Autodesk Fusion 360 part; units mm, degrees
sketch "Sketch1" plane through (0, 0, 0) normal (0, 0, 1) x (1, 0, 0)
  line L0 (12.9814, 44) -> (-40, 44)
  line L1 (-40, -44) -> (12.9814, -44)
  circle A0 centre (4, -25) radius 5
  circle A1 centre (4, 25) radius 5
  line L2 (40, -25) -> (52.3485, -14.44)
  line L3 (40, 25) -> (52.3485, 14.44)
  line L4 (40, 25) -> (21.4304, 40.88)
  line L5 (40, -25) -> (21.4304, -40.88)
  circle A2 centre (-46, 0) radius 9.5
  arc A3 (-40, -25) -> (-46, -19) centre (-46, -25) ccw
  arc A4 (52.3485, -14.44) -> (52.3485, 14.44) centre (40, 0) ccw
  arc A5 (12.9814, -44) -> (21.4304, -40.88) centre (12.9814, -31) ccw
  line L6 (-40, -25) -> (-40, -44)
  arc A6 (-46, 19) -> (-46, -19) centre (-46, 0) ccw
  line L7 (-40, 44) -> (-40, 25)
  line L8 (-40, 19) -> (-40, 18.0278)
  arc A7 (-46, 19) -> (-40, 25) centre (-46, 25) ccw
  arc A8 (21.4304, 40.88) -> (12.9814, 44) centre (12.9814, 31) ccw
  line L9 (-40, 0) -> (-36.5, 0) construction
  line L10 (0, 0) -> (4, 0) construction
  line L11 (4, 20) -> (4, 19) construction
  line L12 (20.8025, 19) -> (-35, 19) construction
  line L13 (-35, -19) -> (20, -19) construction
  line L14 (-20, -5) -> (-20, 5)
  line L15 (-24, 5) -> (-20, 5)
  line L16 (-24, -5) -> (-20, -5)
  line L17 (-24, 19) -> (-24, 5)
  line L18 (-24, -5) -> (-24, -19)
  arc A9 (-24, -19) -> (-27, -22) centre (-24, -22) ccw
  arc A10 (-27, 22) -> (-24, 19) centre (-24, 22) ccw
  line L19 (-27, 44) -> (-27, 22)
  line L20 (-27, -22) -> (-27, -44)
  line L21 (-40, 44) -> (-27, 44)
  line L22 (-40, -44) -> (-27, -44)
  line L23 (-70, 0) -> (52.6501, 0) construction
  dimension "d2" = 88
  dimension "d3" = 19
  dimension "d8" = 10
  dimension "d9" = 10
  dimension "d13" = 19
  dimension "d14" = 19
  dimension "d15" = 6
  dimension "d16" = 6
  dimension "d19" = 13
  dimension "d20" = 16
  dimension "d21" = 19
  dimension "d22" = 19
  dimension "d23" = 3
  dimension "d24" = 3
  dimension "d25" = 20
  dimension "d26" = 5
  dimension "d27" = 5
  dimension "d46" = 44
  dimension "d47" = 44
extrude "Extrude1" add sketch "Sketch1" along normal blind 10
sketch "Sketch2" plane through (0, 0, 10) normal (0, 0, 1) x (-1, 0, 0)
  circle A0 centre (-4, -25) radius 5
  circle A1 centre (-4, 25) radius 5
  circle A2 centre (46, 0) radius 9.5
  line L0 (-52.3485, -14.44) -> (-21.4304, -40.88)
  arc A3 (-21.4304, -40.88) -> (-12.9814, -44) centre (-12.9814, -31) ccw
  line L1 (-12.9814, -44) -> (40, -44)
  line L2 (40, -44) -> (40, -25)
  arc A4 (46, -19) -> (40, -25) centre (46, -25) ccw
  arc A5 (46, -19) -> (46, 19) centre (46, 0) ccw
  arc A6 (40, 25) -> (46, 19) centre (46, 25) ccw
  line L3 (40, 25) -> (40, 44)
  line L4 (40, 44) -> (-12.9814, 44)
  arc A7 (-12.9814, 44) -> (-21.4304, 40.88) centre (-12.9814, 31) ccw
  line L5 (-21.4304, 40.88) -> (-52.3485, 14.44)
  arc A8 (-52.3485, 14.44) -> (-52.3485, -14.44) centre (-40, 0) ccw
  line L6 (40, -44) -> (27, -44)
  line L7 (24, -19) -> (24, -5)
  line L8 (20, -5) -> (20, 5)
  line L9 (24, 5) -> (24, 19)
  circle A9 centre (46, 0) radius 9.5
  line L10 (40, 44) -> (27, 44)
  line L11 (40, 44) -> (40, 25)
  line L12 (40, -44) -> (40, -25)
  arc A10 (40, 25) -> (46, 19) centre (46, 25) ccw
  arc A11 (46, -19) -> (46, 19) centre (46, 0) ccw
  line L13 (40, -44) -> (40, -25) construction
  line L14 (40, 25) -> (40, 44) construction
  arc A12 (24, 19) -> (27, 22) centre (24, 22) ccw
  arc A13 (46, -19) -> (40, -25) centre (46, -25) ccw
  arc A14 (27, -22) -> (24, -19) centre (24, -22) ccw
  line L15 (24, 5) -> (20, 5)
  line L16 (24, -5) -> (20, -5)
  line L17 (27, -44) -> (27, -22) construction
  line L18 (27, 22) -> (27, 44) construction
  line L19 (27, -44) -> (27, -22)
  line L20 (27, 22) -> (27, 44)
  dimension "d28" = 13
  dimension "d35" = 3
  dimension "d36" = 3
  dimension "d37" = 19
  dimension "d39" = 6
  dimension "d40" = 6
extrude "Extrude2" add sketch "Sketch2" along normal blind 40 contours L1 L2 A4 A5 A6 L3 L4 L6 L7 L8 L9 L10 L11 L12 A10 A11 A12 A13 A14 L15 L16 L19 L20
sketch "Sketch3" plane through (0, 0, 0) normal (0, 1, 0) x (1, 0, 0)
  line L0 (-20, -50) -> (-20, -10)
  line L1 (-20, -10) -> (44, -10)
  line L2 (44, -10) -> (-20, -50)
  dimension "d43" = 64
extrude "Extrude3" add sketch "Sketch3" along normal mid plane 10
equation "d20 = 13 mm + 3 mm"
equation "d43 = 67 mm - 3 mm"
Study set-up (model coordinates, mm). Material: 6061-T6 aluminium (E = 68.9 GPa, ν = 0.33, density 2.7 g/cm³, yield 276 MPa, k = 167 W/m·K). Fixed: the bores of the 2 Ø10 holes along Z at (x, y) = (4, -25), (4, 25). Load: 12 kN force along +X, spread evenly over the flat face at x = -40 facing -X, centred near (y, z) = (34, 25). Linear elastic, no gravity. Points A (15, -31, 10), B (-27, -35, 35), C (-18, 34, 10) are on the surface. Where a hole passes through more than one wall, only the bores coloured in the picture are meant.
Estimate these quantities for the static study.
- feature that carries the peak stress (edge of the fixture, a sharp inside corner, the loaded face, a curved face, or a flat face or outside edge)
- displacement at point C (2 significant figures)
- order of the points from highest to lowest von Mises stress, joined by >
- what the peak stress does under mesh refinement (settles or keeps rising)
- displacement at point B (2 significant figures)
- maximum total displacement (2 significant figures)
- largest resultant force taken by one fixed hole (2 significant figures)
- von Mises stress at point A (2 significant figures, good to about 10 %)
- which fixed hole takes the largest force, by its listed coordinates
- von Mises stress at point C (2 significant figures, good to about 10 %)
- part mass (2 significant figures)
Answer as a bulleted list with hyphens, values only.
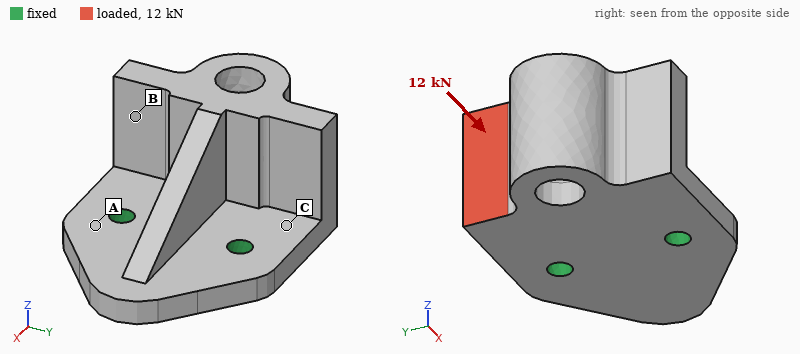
- edge of the fixture
- 0.071 mm
- C > A > B
- keeps rising
- 0.14 mm
- 0.39 mm
- 14 kN
- 50 MPa
- (4, 25)
- 93 MPa
- 440 g
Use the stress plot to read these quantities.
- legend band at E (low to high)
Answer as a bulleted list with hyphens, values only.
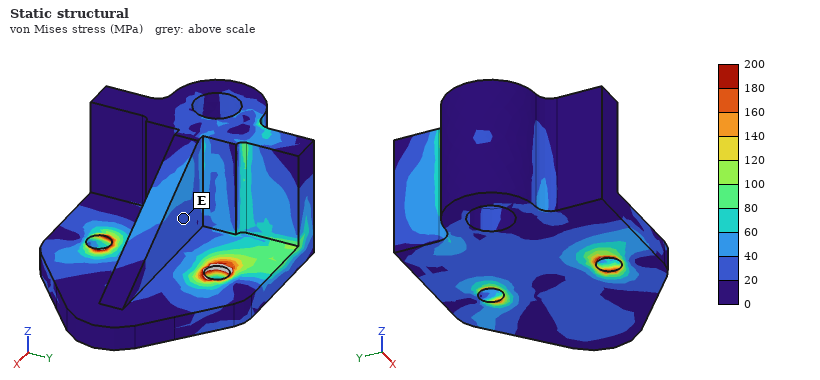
- 20 to 40 MPa
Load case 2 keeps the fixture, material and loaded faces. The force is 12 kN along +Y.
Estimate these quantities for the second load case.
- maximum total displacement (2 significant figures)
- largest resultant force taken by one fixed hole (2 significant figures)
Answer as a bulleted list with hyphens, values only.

- 0.19 mm
- 12 kN
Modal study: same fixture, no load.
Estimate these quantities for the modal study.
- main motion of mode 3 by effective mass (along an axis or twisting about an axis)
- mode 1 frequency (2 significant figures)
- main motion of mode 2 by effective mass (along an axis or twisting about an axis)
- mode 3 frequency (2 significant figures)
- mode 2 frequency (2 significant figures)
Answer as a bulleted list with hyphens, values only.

- along Z
- 1600 Hz
- along Y
- 5400 Hz
- 2800 Hz
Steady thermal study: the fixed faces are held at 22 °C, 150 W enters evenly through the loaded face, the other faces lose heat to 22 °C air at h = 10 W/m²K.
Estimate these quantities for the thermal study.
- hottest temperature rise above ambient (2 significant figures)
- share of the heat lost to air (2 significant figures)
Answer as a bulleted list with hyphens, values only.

- 65 K
- 4.8 %
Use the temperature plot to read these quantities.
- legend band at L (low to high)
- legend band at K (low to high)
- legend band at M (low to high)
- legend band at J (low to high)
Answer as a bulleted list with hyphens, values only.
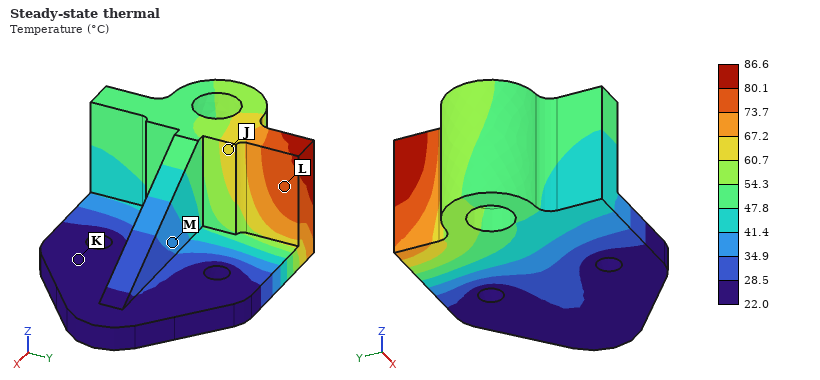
- 73.7 to 80.1 °C
- 22.0 to 28.5 °C
- 34.9 to 41.4 °C
- 60.7 to 67.2 °C
